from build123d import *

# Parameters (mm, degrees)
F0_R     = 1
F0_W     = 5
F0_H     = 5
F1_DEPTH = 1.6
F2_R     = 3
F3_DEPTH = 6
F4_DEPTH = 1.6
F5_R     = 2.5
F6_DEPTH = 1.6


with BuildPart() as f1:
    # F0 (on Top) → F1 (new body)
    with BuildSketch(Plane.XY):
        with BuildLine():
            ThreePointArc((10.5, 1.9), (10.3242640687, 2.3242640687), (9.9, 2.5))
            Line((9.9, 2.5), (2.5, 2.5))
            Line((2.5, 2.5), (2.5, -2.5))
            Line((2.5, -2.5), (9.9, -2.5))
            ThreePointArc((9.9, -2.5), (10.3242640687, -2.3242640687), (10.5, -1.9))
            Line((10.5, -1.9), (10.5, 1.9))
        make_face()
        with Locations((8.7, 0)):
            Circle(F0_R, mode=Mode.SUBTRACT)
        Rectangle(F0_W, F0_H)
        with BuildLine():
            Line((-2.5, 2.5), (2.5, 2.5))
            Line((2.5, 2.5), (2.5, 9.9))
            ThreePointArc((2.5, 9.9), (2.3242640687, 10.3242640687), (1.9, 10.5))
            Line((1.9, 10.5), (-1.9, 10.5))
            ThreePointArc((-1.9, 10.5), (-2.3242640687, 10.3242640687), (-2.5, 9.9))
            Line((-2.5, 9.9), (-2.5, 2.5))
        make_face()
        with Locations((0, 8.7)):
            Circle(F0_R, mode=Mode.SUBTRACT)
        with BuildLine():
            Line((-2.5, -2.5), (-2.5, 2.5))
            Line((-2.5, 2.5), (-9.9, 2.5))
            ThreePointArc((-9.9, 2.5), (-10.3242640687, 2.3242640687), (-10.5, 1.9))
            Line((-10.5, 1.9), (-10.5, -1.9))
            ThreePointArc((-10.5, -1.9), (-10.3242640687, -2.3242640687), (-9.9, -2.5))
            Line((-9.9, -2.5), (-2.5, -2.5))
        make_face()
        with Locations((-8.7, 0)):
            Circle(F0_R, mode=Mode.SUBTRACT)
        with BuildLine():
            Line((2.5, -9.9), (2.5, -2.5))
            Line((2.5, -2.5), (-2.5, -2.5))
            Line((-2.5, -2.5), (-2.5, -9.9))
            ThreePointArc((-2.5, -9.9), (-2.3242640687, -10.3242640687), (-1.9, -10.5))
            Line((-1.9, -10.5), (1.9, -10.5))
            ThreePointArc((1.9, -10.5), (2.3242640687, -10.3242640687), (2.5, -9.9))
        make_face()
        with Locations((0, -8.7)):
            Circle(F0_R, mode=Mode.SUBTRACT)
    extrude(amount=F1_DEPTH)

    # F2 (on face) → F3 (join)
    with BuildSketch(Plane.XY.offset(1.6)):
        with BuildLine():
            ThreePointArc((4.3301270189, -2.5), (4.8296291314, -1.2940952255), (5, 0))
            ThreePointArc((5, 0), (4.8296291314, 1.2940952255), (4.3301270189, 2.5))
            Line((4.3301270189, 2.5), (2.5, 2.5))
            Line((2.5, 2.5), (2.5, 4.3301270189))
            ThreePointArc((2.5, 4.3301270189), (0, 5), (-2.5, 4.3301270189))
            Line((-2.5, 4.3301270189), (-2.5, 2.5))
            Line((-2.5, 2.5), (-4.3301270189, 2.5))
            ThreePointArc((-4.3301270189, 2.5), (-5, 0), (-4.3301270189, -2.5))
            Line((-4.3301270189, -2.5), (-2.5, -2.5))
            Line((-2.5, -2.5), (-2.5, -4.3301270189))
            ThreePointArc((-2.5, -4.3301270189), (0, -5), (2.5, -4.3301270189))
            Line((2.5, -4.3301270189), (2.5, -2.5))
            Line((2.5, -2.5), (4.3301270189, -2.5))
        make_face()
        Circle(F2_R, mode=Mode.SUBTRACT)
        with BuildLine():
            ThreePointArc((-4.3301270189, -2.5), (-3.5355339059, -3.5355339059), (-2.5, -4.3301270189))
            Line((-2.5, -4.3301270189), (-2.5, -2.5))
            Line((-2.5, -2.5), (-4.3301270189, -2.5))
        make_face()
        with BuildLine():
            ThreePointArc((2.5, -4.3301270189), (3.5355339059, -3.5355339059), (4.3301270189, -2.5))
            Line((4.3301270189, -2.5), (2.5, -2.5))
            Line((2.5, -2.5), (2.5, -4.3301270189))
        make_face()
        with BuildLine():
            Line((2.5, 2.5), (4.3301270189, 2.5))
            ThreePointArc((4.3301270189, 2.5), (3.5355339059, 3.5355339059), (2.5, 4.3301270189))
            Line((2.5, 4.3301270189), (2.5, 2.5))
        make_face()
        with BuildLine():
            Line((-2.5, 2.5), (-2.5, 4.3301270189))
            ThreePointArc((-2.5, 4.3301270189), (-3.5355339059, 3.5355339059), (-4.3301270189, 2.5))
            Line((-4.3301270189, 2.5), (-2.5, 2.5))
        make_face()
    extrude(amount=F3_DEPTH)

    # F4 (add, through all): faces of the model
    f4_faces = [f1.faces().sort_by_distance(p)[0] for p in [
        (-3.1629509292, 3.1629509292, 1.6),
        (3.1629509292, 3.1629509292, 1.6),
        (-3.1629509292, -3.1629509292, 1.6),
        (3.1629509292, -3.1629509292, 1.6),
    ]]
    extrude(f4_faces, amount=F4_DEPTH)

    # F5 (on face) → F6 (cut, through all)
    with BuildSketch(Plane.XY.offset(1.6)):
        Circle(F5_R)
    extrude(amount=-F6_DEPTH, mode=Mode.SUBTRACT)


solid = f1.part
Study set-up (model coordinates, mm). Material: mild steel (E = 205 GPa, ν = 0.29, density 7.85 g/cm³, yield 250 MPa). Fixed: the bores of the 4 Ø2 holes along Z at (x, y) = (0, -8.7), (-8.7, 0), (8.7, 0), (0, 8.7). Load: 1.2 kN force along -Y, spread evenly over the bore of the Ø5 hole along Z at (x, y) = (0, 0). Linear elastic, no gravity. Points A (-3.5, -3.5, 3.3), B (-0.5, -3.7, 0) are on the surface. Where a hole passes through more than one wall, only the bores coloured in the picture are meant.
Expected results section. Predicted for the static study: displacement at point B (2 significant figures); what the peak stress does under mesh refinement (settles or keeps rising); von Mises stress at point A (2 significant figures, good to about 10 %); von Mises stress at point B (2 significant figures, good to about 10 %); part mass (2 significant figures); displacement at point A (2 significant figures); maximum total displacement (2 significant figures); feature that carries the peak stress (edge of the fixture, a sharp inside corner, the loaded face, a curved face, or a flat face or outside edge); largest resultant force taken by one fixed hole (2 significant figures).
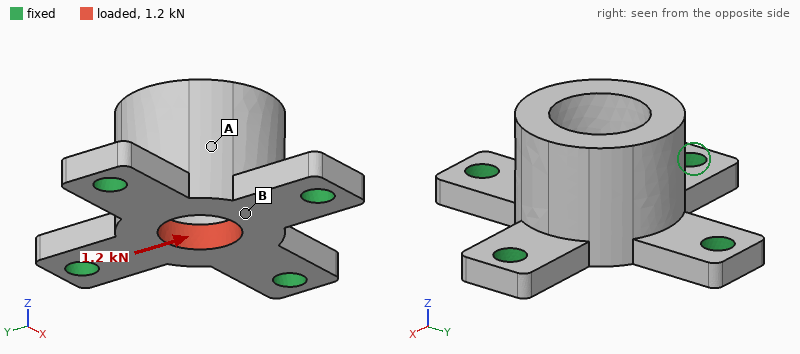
1.4 µm
keeps rising
11 MPa
67 MPa
4.4 g
1.5 µm
2.4 µm
edge of the fixture
490 N
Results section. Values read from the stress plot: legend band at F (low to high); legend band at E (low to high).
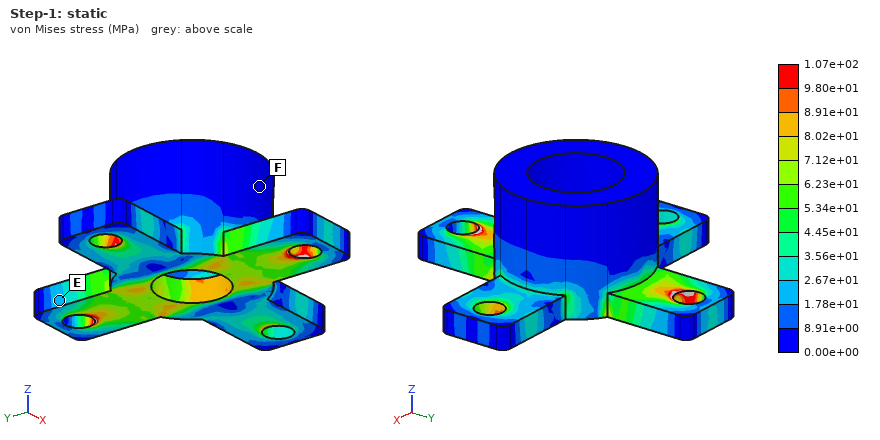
0.00e+00 to 8.91e+00 MPa
1.78e+01 to 2.67e+01 MPa
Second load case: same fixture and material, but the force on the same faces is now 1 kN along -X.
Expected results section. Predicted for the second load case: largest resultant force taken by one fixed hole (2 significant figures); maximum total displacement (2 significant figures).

410 N
2.0 µm
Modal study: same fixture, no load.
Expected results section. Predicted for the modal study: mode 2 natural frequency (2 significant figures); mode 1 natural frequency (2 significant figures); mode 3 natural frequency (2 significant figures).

34 kHz
34 kHz
35 kHz
